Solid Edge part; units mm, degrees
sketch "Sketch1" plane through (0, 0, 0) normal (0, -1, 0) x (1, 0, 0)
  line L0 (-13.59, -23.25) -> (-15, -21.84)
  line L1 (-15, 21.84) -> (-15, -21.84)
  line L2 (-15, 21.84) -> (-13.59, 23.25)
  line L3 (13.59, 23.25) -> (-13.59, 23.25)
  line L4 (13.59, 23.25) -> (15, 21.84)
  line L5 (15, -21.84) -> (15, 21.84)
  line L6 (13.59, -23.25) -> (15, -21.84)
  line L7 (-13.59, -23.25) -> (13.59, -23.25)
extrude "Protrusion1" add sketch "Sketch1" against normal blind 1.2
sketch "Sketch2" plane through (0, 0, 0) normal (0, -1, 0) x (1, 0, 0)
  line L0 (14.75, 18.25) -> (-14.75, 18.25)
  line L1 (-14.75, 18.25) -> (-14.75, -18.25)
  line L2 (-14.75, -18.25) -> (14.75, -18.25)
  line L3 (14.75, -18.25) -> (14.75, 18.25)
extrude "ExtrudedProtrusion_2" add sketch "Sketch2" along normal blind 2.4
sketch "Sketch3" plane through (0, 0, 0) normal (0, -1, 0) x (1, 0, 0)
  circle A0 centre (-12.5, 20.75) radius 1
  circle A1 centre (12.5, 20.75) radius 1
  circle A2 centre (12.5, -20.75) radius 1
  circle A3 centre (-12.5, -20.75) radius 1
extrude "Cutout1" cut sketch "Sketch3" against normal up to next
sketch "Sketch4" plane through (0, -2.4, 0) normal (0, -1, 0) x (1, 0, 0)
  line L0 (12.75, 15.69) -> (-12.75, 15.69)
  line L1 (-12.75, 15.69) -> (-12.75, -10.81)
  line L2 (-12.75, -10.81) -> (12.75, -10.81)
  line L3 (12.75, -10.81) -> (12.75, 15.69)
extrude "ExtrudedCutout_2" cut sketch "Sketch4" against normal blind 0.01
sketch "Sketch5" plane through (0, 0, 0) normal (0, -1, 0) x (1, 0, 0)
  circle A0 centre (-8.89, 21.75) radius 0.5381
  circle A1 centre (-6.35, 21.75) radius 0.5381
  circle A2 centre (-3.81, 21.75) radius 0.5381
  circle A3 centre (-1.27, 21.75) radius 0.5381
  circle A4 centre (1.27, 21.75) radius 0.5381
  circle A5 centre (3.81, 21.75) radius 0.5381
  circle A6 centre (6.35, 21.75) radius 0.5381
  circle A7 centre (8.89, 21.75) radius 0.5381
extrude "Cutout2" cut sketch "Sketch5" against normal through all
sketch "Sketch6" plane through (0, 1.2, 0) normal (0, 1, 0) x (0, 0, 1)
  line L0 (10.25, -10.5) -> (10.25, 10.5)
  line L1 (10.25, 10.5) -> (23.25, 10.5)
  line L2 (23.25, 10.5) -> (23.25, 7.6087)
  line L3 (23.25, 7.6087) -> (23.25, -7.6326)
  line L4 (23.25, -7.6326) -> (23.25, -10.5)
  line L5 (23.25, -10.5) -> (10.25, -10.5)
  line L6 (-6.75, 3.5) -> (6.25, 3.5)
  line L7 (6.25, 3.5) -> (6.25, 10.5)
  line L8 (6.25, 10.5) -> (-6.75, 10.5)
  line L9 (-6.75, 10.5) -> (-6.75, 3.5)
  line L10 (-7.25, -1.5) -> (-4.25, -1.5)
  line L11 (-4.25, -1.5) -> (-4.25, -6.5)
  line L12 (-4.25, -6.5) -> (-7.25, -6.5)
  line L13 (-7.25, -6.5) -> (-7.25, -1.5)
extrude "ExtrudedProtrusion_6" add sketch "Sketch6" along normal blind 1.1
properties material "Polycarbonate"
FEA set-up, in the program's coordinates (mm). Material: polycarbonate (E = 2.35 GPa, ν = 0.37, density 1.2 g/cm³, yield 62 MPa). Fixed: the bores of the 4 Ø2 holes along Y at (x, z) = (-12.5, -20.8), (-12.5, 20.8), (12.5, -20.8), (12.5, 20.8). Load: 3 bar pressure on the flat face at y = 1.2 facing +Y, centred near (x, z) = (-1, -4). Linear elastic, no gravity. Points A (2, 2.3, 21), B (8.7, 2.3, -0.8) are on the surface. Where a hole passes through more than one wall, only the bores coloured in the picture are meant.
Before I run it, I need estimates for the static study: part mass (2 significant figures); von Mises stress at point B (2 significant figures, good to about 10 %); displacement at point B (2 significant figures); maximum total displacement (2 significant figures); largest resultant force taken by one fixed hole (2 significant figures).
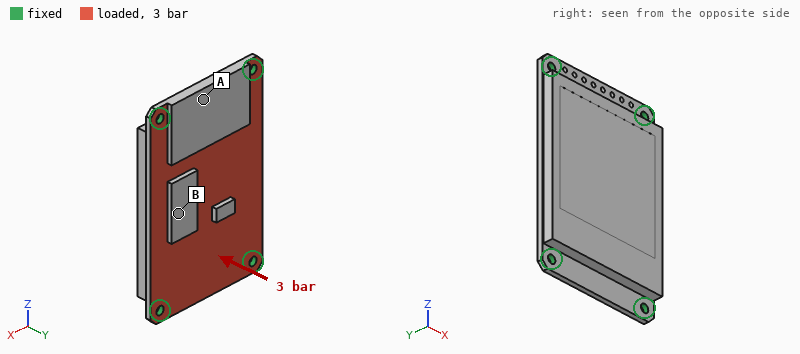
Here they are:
5.6 g
11 MPa
0.49 mm
0.60 mm
160 N
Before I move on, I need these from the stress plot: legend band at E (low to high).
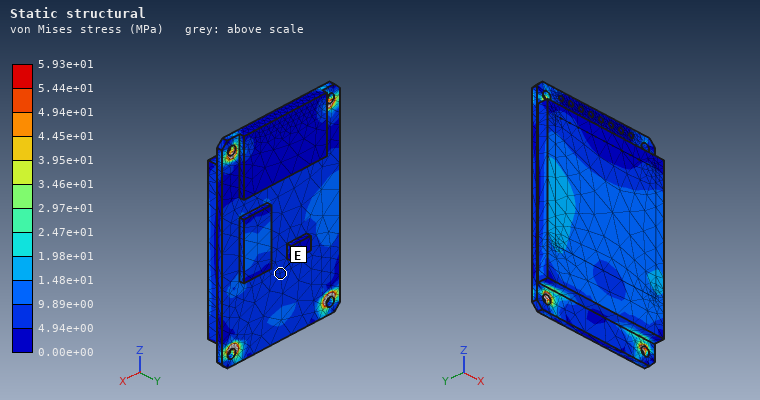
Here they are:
4.94e+00 to 9.89e+00 MPa
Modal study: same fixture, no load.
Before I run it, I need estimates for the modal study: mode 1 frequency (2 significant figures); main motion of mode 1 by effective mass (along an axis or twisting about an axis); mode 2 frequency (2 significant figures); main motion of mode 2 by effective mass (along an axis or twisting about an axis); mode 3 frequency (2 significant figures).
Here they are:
1800 Hz
along Y
3000 Hz
twisting about Z
4100 Hz
